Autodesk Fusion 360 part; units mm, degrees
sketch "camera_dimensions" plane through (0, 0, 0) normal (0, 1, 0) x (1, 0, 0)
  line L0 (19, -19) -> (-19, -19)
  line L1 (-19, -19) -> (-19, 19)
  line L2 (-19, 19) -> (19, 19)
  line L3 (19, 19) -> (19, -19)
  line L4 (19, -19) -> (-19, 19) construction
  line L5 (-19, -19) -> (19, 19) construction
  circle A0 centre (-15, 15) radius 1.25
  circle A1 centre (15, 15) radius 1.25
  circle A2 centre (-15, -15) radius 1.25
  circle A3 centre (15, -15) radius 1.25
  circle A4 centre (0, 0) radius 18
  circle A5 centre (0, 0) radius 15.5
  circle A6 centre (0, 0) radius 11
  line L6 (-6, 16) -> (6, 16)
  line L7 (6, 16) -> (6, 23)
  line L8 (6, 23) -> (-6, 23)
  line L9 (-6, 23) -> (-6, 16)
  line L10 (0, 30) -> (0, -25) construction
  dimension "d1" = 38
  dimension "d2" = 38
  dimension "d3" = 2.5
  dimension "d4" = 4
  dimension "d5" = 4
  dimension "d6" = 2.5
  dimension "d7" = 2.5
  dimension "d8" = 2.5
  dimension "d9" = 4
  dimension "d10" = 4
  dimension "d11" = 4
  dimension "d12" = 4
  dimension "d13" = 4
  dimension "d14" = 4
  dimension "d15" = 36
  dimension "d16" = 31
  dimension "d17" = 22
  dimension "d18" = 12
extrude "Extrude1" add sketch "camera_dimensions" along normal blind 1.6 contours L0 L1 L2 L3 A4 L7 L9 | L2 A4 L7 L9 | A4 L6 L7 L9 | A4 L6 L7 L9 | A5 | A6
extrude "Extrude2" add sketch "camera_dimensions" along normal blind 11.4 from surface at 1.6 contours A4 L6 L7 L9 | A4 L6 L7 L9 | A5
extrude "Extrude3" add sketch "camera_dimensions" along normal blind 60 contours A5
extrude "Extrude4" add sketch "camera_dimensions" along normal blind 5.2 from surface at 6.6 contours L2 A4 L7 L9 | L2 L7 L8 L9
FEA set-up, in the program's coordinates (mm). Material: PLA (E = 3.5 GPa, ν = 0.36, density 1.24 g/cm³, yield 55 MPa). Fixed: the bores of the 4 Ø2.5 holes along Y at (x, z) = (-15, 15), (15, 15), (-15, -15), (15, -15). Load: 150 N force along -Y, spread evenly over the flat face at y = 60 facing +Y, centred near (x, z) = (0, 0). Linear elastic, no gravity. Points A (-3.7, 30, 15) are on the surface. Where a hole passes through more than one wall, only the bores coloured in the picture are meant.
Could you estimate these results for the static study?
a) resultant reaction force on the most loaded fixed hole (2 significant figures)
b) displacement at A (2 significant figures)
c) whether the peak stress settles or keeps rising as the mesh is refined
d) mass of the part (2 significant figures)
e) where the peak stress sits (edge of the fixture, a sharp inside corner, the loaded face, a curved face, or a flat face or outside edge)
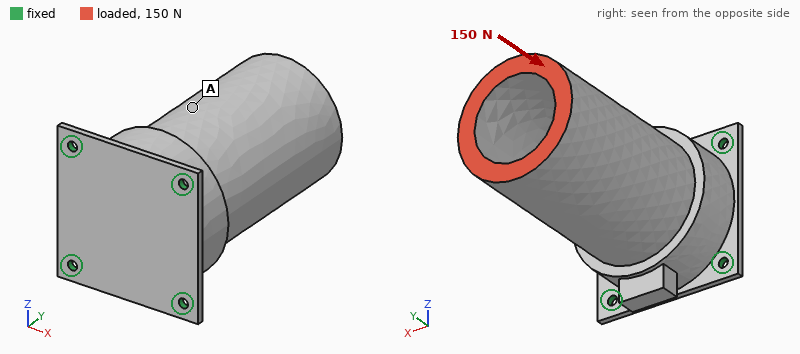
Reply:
42 N
26 µm
keeps rising
34 g
edge of the fixture
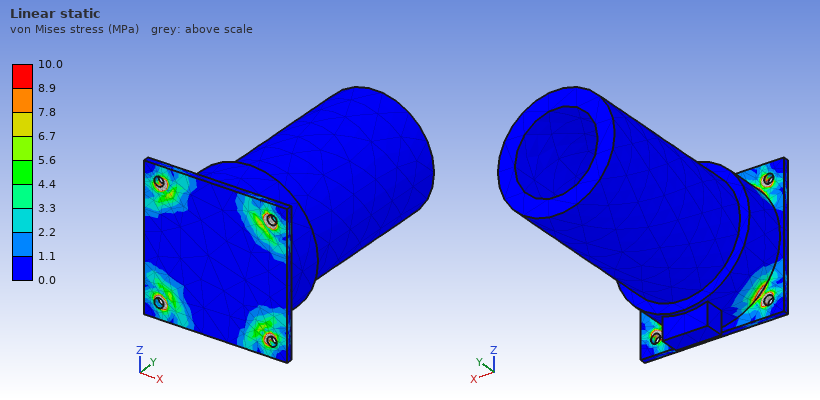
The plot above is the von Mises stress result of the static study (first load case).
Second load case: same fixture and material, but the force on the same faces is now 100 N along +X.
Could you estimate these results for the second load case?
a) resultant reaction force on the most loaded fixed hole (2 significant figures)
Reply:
120 N
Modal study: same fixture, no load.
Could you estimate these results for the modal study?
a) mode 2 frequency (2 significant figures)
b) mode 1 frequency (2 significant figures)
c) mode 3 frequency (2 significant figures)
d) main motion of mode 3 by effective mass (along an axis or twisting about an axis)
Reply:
870 Hz
860 Hz
2100 Hz
along Y
